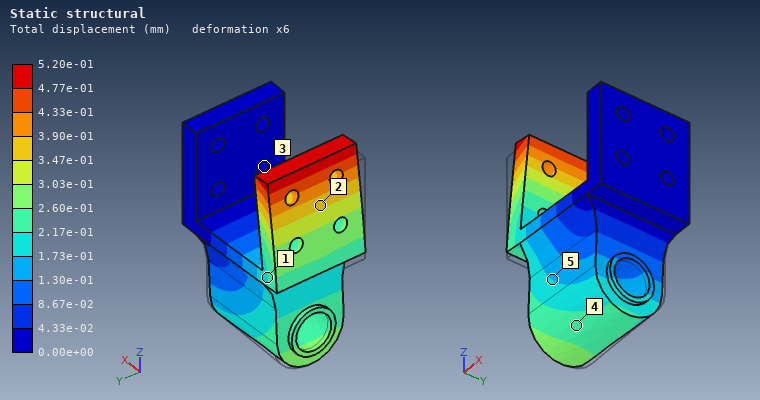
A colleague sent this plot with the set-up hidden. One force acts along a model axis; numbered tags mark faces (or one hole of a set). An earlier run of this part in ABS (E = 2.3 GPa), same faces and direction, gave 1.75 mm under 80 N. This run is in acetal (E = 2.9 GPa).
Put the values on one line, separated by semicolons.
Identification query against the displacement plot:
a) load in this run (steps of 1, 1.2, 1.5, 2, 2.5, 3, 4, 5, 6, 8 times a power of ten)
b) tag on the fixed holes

30 N; 3
